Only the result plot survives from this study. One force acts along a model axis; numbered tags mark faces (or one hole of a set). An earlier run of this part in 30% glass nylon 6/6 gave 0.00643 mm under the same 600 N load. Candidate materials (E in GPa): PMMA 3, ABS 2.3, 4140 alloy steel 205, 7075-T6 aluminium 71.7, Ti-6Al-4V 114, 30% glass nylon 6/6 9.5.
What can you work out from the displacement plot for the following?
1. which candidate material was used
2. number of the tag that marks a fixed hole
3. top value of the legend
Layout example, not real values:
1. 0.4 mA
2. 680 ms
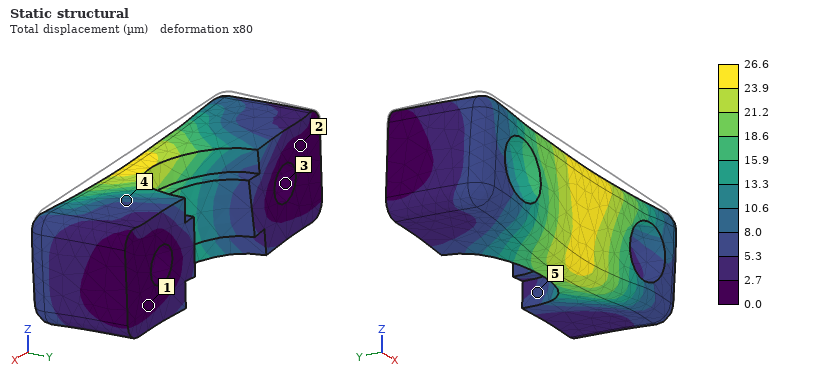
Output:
1. ABS
2. 3
3. 26.6 µm
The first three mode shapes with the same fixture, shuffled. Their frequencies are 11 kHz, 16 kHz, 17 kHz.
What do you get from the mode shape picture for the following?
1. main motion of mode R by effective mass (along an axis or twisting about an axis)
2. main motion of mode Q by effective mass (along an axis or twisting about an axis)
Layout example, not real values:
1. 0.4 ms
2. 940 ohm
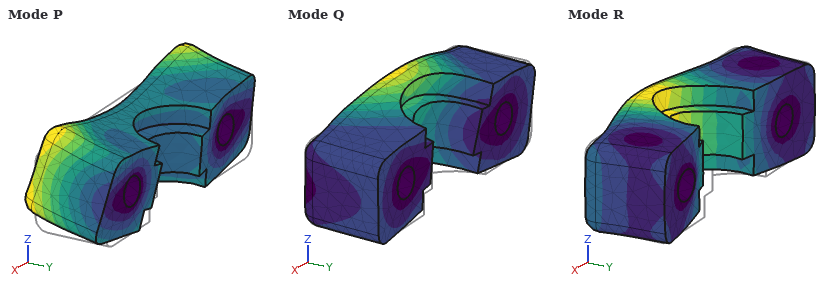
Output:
1. along Y
2. along Z
